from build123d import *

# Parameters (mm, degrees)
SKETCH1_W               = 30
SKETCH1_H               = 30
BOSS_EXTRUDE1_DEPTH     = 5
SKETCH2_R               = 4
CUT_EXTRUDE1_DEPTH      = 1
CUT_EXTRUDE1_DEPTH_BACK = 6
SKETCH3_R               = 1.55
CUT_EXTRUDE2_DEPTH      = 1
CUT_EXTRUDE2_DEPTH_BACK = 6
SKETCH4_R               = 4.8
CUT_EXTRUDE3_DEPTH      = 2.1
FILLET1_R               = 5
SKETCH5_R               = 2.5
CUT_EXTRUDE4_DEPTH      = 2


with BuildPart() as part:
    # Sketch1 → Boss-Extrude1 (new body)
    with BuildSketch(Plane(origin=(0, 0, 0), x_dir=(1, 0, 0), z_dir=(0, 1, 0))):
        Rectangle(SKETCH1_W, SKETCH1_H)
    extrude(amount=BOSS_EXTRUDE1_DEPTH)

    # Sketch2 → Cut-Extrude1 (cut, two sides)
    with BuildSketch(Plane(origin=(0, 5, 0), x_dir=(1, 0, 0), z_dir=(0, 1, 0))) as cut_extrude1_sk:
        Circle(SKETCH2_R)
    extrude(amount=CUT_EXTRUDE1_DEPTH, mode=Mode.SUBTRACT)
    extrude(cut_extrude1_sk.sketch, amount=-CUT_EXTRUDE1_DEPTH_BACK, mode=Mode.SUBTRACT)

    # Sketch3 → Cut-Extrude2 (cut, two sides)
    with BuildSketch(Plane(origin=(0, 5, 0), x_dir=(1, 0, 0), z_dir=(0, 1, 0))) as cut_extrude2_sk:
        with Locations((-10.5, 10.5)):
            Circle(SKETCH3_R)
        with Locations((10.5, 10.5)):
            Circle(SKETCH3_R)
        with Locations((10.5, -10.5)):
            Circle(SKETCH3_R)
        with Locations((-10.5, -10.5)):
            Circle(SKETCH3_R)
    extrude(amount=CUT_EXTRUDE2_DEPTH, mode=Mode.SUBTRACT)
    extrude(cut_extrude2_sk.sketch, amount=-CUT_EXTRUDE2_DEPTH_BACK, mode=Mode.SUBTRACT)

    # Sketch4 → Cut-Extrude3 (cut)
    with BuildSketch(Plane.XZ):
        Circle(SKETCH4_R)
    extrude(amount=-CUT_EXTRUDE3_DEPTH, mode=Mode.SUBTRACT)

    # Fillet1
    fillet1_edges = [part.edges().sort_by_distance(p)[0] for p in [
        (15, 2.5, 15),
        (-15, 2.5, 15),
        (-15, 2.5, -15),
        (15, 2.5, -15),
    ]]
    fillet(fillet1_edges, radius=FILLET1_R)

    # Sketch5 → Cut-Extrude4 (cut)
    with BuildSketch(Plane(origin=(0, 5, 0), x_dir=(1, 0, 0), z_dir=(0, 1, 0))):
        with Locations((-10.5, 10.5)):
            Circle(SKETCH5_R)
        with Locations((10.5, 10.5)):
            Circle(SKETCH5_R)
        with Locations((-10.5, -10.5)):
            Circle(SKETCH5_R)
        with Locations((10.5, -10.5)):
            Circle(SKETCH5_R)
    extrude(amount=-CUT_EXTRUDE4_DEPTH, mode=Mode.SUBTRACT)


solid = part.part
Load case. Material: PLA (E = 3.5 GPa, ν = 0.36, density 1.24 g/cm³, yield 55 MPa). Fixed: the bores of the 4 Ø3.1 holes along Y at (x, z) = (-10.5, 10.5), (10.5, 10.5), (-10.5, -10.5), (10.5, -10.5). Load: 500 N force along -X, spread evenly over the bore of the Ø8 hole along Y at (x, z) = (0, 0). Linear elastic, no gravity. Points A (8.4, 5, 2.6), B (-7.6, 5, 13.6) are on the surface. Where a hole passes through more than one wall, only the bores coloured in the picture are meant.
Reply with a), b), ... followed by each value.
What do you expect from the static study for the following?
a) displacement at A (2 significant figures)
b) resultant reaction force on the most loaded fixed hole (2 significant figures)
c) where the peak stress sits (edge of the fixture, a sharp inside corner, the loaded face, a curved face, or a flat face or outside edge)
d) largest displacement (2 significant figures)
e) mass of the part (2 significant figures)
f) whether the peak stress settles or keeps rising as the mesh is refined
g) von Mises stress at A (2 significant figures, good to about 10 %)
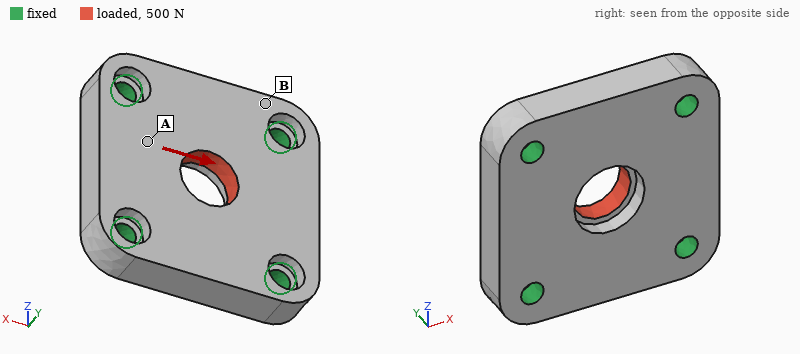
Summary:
a) 16 µm
b) 140 N
c) edge of the fixture
d) 25 µm
e) 4.8 g
f) keeps rising
g) 3.7 MPa
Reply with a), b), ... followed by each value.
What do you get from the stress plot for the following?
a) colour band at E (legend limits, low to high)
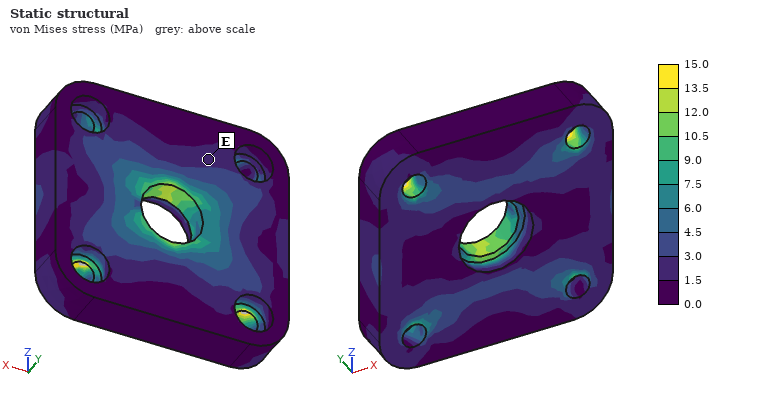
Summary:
a) 1.5 to 3.0 MPa
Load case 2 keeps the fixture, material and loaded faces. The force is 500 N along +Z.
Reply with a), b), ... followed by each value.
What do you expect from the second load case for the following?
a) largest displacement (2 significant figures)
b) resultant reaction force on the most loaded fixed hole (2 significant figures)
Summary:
a) 25 µm
b) 140 N
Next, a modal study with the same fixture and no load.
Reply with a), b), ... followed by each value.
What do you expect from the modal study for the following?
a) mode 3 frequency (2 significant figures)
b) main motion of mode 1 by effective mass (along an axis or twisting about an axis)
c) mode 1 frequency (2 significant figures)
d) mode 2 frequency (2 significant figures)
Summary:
a) 14 kHz
b) along Y
c) 11 kHz
d) 13 kHz
